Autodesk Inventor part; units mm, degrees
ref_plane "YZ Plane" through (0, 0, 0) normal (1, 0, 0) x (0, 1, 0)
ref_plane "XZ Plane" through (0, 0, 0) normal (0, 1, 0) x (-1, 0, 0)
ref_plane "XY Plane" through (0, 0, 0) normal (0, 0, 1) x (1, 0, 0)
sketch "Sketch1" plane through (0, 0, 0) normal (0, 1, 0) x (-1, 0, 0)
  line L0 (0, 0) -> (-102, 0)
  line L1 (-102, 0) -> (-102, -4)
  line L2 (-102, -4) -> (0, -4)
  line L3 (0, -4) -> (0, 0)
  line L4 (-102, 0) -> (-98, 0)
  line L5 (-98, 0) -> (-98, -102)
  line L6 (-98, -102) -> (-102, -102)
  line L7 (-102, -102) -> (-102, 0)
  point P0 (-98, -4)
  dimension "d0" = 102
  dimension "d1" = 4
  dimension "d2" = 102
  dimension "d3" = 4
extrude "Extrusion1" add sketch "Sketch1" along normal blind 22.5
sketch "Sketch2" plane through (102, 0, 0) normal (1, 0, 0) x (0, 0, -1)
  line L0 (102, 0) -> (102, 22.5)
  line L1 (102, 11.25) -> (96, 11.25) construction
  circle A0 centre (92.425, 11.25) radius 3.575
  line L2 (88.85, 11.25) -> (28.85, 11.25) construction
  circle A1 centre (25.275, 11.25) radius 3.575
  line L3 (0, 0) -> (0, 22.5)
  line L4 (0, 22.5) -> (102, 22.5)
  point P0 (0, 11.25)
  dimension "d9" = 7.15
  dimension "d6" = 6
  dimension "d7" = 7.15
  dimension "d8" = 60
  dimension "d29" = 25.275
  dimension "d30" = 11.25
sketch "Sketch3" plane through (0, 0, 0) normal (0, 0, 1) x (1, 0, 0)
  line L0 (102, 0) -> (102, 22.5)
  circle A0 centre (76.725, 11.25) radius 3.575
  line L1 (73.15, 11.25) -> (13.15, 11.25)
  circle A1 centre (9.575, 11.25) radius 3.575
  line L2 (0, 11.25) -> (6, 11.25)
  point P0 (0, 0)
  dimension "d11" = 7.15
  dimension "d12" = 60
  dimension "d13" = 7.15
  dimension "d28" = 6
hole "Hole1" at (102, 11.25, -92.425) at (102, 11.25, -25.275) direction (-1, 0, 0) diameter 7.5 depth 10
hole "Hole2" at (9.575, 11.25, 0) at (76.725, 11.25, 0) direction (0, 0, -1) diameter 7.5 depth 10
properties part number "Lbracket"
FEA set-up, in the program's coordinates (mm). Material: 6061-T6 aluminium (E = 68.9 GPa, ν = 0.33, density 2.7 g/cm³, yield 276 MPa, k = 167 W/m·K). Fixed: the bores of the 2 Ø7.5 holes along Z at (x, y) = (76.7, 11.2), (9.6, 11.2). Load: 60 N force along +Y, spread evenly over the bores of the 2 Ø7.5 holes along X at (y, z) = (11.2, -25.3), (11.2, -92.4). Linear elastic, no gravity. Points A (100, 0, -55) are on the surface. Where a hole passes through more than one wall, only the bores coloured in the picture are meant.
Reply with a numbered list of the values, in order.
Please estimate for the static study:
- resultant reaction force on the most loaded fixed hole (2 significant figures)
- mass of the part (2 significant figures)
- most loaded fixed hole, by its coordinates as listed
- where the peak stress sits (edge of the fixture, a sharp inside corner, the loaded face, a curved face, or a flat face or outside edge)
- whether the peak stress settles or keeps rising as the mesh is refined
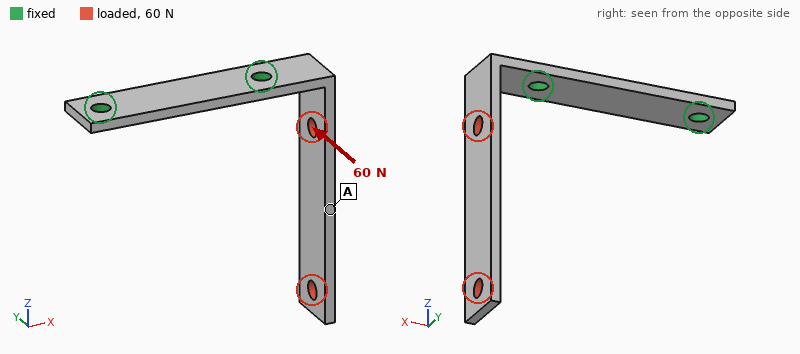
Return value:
1. 68 N
2. 47 g
3. (76.7, 11.2)
4. edge of the fixture
5. keeps rising
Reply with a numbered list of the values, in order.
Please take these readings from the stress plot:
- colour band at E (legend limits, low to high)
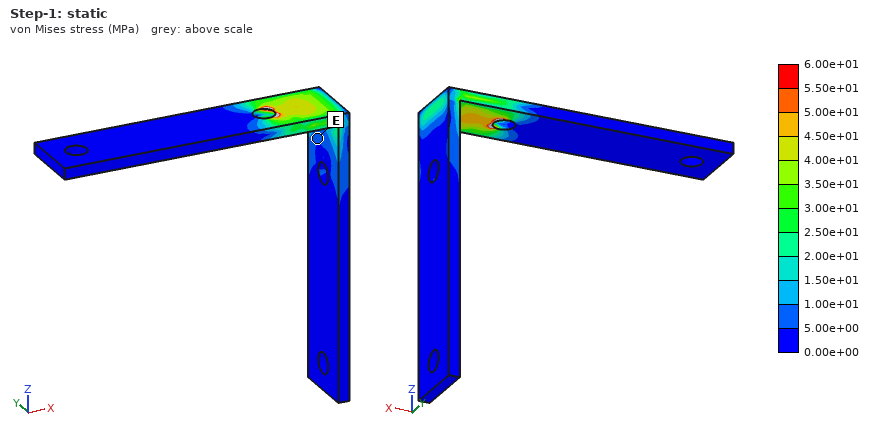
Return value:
1. 5.00e+00 to 1.00e+01 MPa
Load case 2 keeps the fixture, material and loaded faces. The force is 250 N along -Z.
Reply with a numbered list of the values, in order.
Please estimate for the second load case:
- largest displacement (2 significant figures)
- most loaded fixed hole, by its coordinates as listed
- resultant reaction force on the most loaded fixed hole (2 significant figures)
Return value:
1. 0.66 mm
2. (76.7, 11.2)
3. 250 N
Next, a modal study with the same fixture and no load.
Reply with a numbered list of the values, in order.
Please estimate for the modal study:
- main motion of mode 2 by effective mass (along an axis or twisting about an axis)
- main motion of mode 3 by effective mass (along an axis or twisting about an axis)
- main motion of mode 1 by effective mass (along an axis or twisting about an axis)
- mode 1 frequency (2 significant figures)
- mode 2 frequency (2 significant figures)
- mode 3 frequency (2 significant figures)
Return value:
1. along Y
2. along Z
3. along X
4. 250 Hz
5. 460 Hz
6. 1500 Hz
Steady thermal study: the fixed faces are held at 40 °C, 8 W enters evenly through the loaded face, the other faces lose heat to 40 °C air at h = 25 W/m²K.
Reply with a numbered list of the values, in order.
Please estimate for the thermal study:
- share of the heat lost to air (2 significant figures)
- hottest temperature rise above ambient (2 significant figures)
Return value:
1. 34 %
2. 29 K
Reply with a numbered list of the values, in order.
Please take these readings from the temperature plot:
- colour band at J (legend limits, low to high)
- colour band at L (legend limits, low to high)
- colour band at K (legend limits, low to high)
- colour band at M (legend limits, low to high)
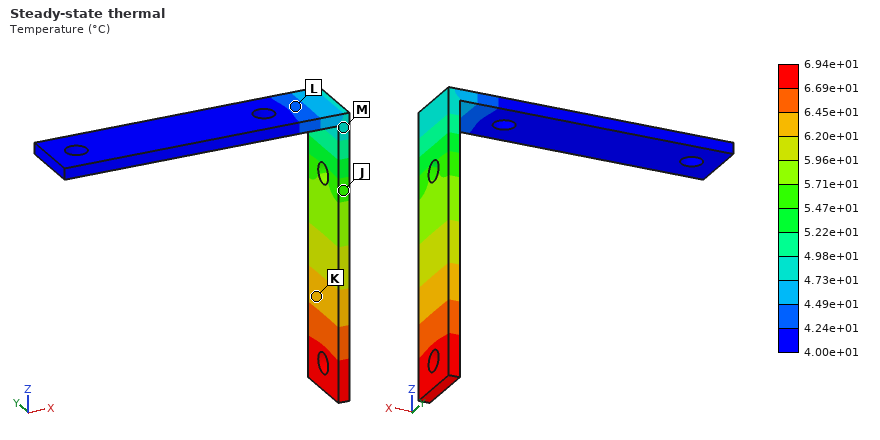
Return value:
1. 5.47e+01 to 5.71e+01 °C
2. 4.24e+01 to 4.49e+01 °C
3. 6.20e+01 to 6.45e+01 °C
4. 4.73e+01 to 4.98e+01 °C
